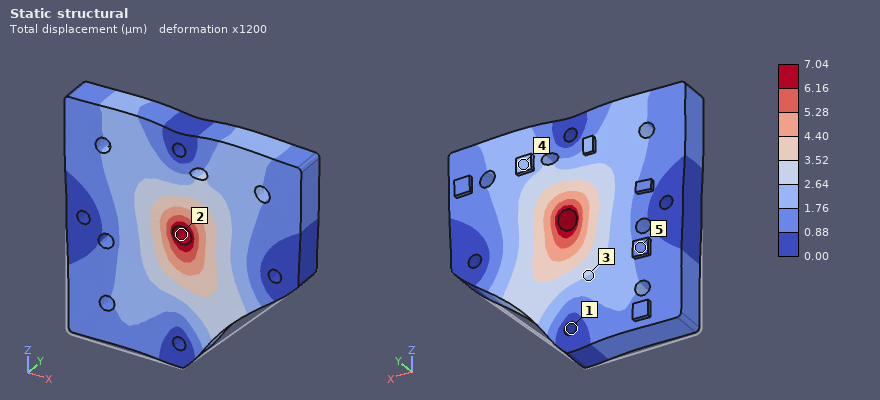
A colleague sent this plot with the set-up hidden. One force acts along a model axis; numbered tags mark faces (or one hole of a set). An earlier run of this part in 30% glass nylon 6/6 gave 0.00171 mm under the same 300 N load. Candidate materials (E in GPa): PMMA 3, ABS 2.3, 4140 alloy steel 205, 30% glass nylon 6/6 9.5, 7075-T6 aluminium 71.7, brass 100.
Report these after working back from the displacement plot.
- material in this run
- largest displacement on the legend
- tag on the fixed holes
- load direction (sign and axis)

ABS
7.04 µm
1
+Z
